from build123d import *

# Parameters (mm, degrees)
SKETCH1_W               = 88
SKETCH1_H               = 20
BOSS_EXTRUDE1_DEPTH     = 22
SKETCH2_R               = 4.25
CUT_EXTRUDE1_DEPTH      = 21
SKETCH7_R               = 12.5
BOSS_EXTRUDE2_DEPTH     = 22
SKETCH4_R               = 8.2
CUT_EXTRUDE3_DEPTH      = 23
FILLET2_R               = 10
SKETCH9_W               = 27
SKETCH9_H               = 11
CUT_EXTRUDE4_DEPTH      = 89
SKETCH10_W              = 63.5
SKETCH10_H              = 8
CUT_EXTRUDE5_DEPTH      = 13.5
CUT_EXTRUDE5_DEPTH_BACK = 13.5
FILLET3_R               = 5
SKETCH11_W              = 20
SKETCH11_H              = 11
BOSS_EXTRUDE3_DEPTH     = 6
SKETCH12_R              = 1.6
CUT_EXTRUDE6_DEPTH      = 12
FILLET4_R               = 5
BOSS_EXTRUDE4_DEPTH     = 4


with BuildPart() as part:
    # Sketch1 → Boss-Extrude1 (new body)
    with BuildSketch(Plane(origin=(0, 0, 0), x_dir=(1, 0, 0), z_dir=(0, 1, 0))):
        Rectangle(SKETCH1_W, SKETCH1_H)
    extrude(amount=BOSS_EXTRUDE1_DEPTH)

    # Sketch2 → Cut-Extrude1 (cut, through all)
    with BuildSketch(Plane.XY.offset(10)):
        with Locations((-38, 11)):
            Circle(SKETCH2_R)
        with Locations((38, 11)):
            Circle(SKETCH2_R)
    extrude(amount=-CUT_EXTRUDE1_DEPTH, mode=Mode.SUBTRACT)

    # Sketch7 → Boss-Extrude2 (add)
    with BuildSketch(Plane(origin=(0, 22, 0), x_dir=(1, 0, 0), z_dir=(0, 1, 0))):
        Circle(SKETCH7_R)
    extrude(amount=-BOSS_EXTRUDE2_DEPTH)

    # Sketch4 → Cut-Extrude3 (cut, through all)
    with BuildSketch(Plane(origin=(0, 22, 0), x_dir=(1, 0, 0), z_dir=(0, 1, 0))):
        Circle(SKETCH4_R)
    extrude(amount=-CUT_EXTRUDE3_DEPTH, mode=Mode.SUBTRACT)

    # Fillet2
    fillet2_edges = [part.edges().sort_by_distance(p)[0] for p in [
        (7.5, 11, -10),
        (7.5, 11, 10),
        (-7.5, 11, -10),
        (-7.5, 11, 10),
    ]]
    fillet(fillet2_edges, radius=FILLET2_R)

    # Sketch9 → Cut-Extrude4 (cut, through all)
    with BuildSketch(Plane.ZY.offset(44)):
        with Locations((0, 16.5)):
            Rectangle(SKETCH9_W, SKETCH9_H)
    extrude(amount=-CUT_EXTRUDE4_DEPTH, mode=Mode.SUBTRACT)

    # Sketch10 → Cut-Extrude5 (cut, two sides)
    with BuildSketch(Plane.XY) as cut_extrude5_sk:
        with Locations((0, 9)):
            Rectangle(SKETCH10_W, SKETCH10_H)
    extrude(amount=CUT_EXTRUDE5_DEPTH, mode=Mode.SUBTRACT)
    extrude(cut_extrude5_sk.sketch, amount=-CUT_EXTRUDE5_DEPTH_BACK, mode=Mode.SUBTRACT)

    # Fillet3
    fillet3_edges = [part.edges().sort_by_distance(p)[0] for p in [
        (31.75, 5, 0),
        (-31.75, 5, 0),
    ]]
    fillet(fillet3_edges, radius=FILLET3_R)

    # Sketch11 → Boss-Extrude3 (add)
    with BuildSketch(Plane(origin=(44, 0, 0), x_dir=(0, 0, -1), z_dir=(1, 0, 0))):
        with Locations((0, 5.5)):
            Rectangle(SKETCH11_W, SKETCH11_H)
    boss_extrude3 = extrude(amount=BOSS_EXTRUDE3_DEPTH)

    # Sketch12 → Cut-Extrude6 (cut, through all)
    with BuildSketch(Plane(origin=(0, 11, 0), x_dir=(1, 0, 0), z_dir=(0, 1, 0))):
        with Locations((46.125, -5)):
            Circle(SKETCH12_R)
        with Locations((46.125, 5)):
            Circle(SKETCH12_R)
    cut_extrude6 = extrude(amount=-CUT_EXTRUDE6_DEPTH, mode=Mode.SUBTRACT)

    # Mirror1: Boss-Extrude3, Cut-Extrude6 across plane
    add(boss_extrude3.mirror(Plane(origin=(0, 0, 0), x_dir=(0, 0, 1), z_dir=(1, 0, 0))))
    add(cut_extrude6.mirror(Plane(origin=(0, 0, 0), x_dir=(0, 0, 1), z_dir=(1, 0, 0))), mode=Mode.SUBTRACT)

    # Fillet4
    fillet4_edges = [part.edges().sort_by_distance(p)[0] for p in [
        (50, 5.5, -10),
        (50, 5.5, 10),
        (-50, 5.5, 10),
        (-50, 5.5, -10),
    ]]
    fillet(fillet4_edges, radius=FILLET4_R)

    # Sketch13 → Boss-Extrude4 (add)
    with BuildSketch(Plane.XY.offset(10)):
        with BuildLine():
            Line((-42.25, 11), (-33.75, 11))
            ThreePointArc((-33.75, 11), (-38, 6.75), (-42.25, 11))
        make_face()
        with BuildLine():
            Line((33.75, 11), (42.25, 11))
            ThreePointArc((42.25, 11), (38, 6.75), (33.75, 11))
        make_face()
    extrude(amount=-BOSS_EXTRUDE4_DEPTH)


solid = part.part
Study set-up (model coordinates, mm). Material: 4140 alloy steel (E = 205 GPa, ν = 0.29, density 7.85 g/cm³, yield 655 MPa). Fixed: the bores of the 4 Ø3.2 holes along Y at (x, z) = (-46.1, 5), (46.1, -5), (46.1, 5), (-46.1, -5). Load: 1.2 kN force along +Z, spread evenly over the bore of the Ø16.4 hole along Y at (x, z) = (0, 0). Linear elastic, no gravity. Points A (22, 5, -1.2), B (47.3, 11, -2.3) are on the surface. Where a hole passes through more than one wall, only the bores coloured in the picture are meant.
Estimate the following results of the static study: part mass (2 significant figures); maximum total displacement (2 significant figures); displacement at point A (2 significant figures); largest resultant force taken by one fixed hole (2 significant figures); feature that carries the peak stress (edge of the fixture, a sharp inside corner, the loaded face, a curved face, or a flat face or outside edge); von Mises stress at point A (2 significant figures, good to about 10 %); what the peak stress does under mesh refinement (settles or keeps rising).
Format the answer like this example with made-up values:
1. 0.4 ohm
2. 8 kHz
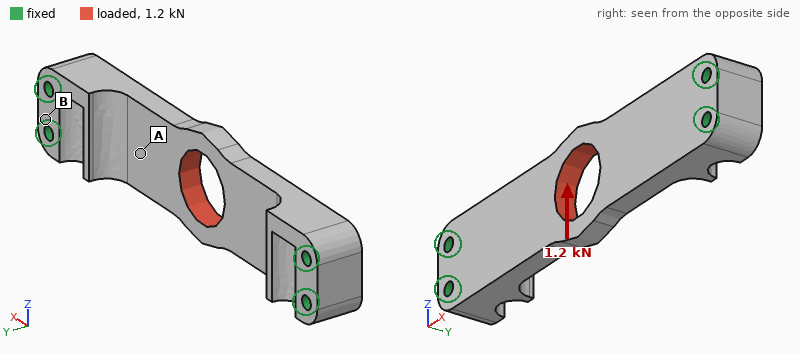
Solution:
1. 97 g
2. 8.8 µm
3. 4.8 µm
4. 1.2 kN
5. edge of the fixture
6. 16 MPa
7. keeps rising
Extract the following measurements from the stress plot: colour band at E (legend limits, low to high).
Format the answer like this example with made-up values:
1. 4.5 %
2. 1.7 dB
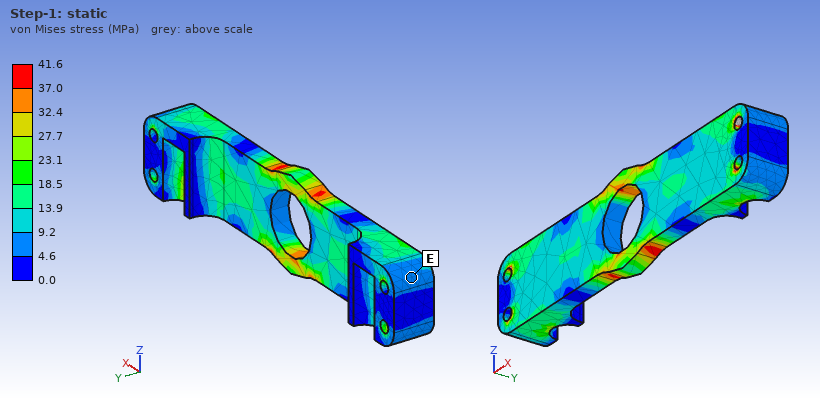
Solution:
1. 4.6 to 9.2 MPa
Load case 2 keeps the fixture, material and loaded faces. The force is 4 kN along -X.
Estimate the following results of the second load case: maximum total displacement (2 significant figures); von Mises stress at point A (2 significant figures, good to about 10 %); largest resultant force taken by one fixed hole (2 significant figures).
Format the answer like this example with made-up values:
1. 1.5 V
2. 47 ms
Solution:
1. 4.8 µm
2. 26 MPa
3. 1.0 kN
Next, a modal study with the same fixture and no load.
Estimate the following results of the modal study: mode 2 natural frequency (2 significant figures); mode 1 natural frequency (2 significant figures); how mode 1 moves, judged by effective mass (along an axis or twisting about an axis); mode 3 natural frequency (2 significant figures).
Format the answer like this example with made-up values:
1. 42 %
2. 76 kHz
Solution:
1. 11 kHz
2. 5000 Hz
3. along Y
4. 11 kHz
